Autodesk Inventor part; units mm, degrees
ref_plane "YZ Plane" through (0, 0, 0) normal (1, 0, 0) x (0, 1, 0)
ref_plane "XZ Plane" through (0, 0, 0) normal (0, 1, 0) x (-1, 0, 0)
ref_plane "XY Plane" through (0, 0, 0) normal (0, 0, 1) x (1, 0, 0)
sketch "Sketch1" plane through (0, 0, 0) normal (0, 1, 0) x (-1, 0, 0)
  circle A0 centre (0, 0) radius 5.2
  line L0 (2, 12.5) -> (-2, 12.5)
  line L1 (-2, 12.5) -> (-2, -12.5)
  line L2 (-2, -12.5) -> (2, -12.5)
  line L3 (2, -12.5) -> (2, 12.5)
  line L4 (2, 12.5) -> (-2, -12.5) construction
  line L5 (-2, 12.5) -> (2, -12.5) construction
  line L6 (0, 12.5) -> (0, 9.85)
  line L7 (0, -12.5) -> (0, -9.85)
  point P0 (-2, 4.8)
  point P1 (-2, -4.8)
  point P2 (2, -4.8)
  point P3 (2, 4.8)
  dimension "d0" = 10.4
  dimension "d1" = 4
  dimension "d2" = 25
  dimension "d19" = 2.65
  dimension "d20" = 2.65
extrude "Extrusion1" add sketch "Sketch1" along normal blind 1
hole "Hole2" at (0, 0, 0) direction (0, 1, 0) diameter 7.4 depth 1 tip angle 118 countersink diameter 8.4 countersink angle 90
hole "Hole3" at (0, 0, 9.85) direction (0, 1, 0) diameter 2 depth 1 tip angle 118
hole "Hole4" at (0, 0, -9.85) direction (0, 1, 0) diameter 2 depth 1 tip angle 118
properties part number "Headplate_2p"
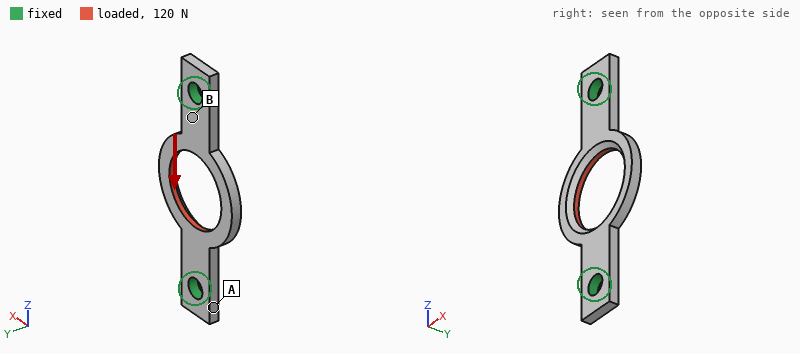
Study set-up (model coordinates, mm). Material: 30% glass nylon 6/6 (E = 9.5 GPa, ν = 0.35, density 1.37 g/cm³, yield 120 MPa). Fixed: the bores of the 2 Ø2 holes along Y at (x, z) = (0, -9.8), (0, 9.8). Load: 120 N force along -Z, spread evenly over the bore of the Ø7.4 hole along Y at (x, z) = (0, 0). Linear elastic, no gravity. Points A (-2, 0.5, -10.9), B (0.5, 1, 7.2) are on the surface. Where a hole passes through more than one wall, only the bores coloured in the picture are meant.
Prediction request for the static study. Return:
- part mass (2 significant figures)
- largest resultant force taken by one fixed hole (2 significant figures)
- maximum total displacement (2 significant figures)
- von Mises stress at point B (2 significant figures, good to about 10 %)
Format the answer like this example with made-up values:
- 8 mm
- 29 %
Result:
- 0.13 g
- 60 N
- 34 µm
- 17 MPa
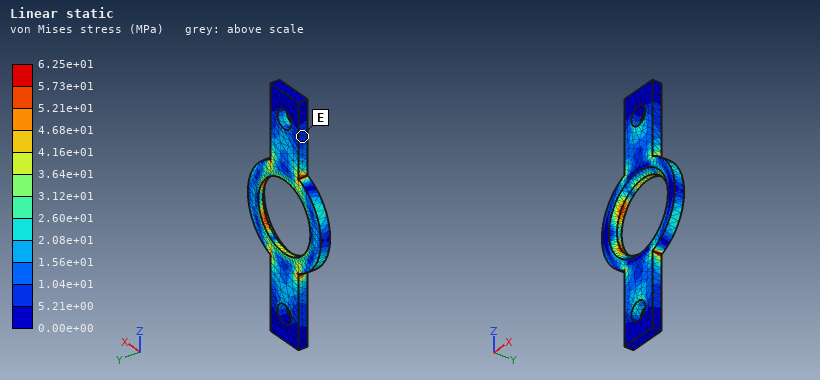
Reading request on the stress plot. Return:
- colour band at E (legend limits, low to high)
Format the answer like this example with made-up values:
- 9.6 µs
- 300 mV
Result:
- 5.21e+00 to 1.04e+01 MPa
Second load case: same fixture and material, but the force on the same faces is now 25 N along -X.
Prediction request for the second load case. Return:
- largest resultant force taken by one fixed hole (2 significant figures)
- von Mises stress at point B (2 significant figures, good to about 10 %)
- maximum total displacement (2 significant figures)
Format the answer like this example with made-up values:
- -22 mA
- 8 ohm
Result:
- 13 N
- 12 MPa
- 33 µm
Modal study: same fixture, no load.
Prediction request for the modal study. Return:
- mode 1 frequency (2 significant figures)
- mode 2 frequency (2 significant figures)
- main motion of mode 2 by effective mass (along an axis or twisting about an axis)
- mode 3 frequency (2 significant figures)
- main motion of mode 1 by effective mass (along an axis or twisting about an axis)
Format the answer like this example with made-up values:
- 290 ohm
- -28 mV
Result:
- 7100 Hz
- 7600 Hz
- twisting about Z
- 17 kHz
- along Y
